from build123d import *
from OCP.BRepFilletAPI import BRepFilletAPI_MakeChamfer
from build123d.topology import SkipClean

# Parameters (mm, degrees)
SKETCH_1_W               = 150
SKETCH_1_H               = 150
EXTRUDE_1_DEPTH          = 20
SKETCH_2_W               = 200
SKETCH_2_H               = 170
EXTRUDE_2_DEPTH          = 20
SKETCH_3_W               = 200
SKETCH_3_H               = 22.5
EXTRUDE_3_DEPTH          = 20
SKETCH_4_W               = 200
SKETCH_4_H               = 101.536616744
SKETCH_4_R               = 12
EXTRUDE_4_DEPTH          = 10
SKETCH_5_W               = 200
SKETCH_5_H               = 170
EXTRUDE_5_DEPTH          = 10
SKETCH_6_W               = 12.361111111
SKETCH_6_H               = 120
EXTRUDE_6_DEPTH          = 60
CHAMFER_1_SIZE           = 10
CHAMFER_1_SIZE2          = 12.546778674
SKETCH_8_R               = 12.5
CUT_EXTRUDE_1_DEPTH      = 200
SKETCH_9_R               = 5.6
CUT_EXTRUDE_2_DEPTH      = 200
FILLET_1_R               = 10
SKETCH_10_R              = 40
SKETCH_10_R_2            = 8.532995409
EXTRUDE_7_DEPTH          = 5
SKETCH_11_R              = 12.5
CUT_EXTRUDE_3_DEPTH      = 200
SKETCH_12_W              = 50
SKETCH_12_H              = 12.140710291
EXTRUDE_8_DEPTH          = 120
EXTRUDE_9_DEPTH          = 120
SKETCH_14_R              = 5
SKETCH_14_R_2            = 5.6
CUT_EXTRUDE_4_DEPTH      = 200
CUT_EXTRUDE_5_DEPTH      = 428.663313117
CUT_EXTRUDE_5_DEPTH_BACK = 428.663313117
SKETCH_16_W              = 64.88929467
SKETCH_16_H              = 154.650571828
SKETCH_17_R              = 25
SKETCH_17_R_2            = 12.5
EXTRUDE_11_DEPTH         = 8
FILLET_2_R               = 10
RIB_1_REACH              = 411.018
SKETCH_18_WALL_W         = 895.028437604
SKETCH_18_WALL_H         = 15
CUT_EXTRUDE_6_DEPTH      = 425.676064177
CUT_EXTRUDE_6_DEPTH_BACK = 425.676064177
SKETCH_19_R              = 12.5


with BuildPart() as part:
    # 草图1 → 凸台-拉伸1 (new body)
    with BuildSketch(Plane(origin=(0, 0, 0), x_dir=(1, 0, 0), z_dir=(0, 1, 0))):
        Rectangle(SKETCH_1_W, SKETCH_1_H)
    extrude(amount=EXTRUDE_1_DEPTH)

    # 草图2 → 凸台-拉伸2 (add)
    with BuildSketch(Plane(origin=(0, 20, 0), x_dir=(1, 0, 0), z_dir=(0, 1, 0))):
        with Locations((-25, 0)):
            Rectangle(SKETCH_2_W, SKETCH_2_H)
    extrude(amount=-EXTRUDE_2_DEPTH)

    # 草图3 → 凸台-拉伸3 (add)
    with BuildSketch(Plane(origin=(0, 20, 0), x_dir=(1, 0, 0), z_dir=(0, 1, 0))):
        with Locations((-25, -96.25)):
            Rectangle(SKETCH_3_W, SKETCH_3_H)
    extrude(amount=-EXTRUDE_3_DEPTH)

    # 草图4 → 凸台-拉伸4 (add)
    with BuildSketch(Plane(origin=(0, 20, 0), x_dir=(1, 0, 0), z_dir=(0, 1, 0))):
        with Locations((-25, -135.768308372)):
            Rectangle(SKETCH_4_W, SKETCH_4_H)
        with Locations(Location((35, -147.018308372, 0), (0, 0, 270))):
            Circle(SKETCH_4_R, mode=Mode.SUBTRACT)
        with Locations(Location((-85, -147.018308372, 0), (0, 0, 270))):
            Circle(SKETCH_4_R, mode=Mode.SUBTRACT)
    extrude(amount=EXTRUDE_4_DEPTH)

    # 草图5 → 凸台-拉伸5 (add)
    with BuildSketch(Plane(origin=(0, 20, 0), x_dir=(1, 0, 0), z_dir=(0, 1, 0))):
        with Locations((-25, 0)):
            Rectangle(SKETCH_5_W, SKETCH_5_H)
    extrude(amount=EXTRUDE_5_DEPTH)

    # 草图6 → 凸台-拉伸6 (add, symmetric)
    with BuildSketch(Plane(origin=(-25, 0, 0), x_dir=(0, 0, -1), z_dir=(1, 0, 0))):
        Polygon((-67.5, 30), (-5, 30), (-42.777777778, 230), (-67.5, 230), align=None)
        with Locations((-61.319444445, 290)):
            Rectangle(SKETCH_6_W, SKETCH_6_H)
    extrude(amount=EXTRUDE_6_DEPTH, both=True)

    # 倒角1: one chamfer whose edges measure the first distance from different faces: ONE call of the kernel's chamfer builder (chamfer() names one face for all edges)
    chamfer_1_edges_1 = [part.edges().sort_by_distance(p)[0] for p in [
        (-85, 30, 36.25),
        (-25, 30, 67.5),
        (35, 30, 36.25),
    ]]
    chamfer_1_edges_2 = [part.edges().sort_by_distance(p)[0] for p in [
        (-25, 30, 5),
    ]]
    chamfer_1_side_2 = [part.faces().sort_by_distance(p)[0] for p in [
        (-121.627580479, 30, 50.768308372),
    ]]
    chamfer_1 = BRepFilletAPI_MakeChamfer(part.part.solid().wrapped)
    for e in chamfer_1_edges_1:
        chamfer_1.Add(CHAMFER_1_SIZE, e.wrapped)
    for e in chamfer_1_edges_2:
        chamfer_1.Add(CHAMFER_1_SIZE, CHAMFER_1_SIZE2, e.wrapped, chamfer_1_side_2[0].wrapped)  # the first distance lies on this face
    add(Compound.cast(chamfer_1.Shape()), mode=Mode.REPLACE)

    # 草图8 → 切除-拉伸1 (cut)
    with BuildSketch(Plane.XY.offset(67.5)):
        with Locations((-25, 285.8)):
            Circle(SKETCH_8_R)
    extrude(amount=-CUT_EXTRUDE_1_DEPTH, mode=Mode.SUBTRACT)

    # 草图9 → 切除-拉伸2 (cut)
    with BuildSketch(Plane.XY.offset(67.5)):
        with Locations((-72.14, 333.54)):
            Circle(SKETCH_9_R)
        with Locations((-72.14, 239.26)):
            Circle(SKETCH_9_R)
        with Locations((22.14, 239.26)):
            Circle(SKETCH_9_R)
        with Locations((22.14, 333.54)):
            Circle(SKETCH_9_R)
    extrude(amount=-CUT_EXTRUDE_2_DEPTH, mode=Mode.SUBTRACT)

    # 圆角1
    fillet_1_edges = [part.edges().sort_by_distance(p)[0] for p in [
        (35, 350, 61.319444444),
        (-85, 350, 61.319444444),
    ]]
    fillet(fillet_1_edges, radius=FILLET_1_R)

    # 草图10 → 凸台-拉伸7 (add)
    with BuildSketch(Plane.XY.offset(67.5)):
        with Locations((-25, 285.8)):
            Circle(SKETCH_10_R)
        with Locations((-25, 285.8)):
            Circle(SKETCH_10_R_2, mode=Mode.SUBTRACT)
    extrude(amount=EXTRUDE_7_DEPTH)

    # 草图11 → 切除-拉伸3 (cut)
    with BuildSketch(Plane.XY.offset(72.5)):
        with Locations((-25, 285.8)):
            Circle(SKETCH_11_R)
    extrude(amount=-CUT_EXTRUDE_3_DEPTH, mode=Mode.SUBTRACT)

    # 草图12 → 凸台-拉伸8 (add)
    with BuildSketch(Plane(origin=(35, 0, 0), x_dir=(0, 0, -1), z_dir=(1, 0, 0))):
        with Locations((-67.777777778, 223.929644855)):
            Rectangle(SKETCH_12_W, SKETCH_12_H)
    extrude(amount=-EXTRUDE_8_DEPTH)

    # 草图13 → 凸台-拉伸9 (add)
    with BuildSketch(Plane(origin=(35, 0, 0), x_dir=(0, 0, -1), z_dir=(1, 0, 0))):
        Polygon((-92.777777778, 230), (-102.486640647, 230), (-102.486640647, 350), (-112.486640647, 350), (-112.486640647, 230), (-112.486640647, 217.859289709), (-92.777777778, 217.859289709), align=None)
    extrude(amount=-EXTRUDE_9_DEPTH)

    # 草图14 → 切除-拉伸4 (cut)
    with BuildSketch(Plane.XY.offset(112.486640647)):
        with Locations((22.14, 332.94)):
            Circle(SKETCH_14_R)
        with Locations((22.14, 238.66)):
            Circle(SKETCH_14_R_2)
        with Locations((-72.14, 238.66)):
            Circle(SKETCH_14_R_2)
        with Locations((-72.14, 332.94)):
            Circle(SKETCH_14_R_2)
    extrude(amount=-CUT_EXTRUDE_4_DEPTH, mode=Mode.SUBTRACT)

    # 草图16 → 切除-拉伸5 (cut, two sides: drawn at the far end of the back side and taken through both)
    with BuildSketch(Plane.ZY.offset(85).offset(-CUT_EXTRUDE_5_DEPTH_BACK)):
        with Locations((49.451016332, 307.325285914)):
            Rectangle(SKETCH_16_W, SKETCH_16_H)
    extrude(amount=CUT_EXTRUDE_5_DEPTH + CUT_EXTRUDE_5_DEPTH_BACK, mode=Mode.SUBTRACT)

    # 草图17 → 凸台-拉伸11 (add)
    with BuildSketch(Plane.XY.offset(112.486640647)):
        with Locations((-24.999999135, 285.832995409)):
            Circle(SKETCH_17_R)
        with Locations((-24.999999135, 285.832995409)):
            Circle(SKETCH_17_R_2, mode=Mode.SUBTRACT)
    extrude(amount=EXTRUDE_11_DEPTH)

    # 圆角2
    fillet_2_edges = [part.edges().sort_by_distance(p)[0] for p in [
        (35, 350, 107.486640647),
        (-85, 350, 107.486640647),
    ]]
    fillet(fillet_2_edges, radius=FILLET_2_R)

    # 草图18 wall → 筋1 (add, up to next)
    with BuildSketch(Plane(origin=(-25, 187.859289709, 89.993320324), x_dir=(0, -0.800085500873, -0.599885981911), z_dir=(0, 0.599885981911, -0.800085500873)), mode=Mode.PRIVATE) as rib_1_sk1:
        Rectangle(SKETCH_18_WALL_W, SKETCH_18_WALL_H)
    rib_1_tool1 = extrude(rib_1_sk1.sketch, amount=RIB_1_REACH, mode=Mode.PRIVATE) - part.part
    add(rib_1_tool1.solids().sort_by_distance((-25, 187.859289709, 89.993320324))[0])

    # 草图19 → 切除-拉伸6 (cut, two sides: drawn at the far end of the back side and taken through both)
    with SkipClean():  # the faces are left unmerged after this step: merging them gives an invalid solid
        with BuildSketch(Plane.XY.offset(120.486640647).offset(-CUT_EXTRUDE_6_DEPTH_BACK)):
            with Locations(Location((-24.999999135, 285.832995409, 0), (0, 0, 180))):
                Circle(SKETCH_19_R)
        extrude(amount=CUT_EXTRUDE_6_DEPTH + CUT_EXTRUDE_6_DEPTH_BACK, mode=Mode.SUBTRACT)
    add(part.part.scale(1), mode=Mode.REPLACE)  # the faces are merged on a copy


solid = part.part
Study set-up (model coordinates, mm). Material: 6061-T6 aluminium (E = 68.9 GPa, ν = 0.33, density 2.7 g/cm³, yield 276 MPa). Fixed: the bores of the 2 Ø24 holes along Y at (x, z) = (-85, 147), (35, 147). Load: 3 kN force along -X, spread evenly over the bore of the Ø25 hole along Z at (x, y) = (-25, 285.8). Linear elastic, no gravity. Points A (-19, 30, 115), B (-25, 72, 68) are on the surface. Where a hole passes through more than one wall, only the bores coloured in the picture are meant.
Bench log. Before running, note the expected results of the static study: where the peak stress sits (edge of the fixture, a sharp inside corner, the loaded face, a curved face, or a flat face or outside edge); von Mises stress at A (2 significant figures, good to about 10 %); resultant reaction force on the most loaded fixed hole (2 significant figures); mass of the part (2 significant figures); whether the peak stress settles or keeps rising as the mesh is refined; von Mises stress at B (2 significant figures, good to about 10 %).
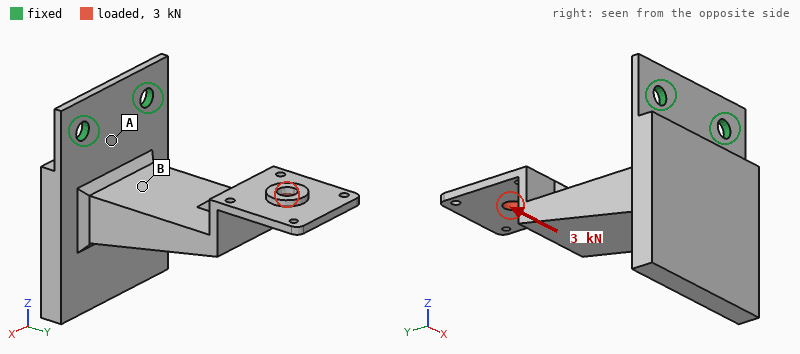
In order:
edge of the fixture
16 MPa
6.1 kN
7.0 kg
keeps rising
6.8 MPa
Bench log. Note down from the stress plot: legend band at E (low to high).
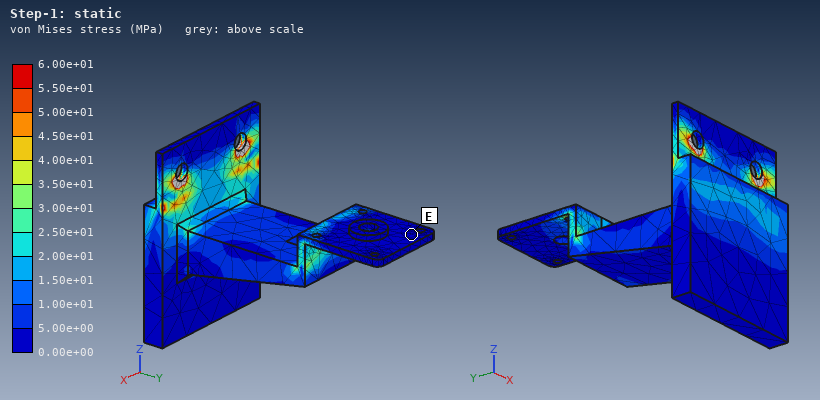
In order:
0.00e+00 to 5.00e+00 MPa
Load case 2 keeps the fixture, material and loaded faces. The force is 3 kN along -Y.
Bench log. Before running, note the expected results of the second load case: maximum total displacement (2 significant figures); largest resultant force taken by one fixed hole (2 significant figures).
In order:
0.31 mm
1.5 kN
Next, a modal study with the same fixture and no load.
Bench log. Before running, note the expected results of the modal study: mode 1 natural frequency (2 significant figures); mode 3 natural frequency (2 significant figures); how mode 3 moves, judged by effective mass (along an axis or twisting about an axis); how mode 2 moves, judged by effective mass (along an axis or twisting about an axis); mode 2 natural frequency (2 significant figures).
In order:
75 Hz
460 Hz
along Y
along X
320 Hz
